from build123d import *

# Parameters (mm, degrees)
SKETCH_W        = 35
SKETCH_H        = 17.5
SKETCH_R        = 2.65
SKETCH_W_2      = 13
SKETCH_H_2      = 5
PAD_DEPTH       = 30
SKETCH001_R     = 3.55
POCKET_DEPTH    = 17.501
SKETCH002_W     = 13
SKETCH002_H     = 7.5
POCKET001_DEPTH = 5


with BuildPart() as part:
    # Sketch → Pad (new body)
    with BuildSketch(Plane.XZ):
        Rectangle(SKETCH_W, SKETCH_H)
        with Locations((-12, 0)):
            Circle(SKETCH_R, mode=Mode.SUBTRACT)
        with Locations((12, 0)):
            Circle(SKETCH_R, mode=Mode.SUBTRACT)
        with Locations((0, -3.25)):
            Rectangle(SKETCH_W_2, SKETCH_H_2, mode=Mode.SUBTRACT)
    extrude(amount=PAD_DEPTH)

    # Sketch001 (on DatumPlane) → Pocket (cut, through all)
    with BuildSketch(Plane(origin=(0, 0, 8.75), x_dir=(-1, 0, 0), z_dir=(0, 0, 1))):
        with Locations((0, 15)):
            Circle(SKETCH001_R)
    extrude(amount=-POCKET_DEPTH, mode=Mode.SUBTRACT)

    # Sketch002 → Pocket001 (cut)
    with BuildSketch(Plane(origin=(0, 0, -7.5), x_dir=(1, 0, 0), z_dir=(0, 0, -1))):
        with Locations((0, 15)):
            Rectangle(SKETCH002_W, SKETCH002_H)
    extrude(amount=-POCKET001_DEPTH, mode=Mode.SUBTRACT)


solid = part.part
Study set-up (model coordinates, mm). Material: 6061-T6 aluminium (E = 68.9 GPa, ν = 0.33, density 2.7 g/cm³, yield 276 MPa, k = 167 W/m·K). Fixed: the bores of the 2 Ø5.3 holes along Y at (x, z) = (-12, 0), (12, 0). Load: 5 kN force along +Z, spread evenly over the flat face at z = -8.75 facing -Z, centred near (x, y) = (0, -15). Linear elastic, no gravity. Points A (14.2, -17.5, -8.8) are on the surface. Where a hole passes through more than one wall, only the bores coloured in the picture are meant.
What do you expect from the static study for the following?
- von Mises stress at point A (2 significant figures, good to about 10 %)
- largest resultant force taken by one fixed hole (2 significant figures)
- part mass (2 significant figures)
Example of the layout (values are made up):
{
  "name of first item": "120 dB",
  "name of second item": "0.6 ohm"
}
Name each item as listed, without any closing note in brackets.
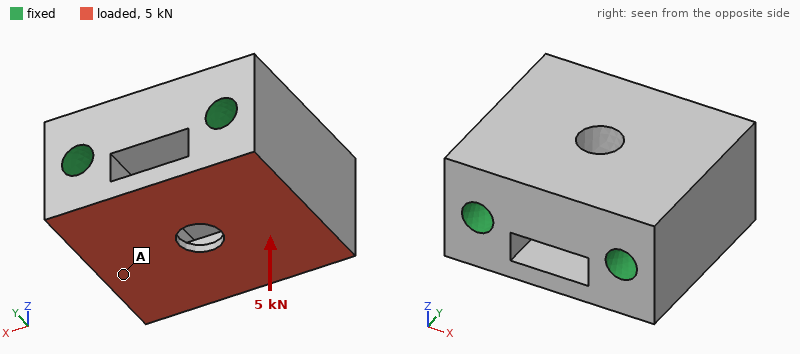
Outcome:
{
  "von Mises stress at point A": "6.5 MPa",
  "largest resultant force taken by one fixed hole": "2.5 kN",
  "part mass": "39 g"
}
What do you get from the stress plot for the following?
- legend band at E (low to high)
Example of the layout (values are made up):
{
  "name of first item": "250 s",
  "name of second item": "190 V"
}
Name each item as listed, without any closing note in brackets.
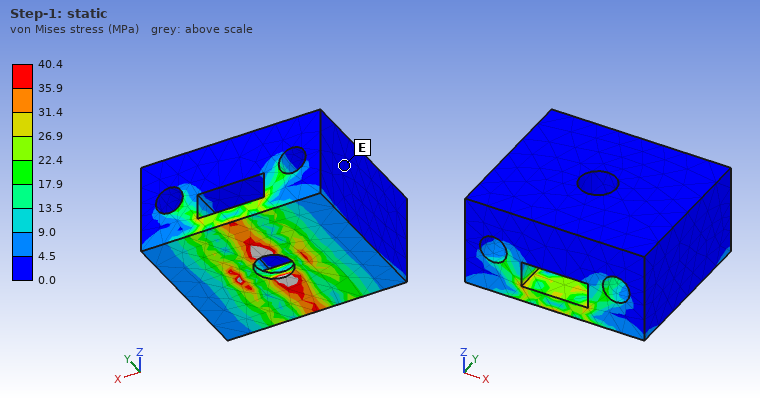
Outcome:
{
  "legend band at E": "0.0 to 4.5 MPa"
}
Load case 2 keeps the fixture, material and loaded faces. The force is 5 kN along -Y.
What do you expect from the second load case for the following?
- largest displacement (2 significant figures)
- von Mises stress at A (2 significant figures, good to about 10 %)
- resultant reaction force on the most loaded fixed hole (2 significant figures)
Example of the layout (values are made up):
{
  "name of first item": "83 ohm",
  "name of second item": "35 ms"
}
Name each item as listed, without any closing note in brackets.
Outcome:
{
  "largest displacement": "7.8 µm",
  "von Mises stress at A": "9.0 MPa",
  "resultant reaction force on the most loaded fixed hole": "2.5 kN"
}
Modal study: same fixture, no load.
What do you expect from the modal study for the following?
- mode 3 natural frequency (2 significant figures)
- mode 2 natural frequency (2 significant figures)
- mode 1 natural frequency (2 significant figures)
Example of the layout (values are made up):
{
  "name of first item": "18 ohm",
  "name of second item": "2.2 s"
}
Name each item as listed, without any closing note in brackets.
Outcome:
{
  "mode 3 natural frequency": "60 kHz",
  "mode 2 natural frequency": "51 kHz",
  "mode 1 natural frequency": "49 kHz"
}
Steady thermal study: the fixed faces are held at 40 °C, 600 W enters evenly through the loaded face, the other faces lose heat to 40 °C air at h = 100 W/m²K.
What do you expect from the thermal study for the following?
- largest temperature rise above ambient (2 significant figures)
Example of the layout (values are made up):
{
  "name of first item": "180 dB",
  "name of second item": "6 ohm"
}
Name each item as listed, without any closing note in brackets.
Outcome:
{
  "largest temperature rise above ambient": "75 K"
}
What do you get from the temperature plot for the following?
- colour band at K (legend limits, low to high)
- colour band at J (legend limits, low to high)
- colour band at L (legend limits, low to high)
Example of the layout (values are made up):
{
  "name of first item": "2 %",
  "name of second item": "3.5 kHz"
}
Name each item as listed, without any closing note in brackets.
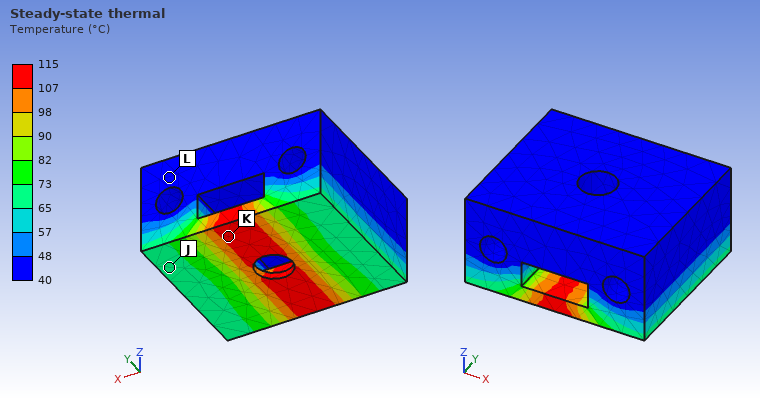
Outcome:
{
  "colour band at K": "107 to 115 °C",
  "colour band at J": "65 to 73 °C",
  "colour band at L": "40 to 48 °C"
}
